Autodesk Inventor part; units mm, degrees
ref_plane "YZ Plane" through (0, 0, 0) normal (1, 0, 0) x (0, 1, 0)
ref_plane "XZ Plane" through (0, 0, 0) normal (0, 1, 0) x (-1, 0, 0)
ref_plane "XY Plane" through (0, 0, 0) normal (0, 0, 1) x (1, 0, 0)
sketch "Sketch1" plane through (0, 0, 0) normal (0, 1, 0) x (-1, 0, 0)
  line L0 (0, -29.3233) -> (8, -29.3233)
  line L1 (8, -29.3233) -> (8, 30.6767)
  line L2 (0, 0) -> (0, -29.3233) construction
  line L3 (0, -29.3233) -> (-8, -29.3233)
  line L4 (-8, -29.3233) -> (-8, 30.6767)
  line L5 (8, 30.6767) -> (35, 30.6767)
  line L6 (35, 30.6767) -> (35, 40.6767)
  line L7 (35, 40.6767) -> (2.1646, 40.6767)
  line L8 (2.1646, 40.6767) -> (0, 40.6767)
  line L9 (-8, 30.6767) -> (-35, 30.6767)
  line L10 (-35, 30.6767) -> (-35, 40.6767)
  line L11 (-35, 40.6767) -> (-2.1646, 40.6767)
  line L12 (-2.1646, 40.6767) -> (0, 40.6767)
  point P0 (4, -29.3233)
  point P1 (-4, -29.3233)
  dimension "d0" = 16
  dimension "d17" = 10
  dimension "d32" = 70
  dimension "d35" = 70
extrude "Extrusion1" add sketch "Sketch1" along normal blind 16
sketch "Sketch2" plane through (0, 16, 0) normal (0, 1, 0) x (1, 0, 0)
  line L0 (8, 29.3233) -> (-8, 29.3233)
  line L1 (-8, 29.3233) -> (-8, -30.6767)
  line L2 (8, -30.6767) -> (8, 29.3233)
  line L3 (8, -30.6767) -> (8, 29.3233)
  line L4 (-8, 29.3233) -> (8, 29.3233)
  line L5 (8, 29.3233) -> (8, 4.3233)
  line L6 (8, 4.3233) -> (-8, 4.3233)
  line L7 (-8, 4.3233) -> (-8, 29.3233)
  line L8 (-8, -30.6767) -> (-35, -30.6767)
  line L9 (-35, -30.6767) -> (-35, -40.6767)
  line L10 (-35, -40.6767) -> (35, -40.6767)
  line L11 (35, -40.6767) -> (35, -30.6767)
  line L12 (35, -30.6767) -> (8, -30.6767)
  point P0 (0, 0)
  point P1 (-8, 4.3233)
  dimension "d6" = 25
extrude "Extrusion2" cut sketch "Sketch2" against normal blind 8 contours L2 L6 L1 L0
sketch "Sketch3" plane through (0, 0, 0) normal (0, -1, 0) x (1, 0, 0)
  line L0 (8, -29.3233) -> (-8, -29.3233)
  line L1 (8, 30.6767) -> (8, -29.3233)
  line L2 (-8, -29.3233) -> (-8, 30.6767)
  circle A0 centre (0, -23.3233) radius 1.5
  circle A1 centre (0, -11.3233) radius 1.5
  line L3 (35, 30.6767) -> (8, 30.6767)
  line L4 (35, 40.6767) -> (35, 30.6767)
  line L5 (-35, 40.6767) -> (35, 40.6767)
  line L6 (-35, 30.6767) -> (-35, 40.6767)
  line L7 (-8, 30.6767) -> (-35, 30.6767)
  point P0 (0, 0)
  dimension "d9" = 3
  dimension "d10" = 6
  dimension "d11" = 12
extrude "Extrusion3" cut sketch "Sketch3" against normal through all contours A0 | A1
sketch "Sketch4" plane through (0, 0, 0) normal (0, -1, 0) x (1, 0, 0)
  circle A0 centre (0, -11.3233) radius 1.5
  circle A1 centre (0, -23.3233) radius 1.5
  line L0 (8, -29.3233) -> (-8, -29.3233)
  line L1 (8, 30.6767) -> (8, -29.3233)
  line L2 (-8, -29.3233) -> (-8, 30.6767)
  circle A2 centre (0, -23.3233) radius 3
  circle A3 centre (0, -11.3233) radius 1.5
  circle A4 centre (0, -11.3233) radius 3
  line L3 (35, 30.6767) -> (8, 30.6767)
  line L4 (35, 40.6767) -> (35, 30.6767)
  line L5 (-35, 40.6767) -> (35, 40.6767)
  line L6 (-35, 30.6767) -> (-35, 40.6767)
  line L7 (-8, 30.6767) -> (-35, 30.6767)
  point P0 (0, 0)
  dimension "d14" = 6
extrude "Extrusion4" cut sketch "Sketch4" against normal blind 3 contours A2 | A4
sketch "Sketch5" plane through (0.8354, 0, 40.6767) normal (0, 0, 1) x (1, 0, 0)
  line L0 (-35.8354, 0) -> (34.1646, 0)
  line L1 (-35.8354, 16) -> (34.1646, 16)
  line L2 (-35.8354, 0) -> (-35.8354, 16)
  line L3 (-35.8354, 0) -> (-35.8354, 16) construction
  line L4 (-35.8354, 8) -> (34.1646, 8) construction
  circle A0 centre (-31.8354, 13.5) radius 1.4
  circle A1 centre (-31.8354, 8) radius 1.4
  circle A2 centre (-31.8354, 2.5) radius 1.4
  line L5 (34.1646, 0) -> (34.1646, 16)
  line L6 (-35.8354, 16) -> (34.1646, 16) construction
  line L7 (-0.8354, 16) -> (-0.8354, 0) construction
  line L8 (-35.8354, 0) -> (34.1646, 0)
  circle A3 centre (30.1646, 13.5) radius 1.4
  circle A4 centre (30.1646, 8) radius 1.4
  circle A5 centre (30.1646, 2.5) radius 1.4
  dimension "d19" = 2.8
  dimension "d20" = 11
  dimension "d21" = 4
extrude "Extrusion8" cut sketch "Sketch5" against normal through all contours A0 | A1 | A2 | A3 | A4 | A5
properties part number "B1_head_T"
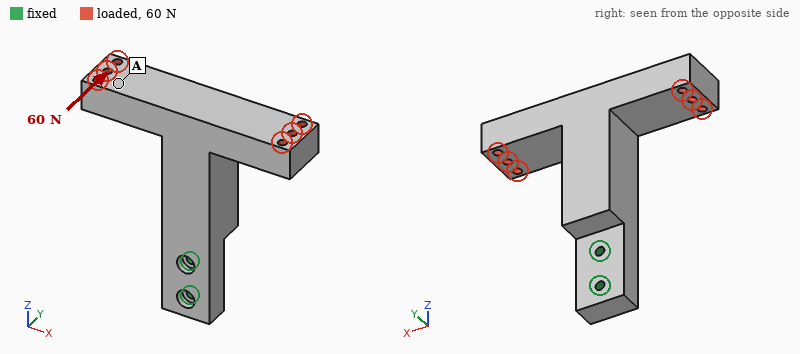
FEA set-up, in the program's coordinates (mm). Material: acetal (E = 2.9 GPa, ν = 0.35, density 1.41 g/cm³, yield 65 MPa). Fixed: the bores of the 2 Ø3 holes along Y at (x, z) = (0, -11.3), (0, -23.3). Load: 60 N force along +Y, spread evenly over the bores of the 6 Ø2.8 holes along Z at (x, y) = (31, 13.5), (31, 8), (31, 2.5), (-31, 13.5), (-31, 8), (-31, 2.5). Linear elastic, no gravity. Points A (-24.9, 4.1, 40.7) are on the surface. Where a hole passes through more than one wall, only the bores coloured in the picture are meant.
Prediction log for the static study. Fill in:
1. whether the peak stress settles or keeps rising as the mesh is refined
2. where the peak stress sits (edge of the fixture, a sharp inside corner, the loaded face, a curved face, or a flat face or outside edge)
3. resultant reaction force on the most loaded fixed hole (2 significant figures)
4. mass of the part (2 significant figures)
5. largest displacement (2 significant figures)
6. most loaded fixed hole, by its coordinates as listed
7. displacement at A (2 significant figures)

keeps rising
edge of the fixture
220 N
32 g
1.1 mm
(0, -11.3)
1.0 mm
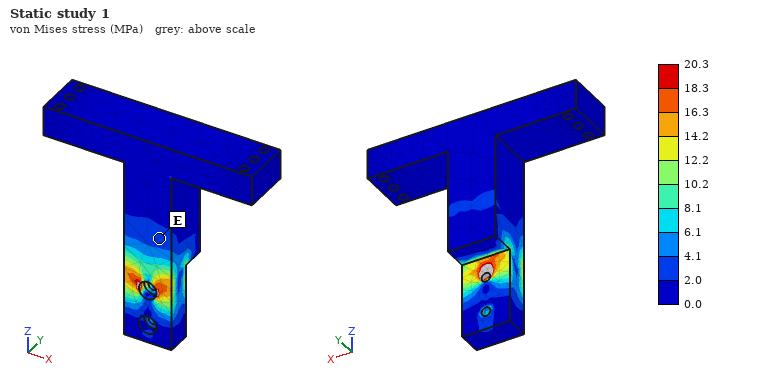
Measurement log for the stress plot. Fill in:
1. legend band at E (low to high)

2.0 to 4.1 MPa
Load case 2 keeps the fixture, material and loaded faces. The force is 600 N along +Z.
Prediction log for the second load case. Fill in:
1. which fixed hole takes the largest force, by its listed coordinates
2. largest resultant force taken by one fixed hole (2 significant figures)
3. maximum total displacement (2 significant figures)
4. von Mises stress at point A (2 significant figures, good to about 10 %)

(0, -11.3)
530 N
1.2 mm
7.0 MPa
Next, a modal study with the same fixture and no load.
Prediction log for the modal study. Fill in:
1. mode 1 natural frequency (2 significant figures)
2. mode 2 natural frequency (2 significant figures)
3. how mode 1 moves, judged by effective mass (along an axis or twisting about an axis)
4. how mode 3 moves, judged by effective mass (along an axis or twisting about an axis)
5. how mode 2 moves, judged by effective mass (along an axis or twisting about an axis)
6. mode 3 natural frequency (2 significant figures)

290 Hz
420 Hz
along Y
twisting about Z
along X
590 Hz
